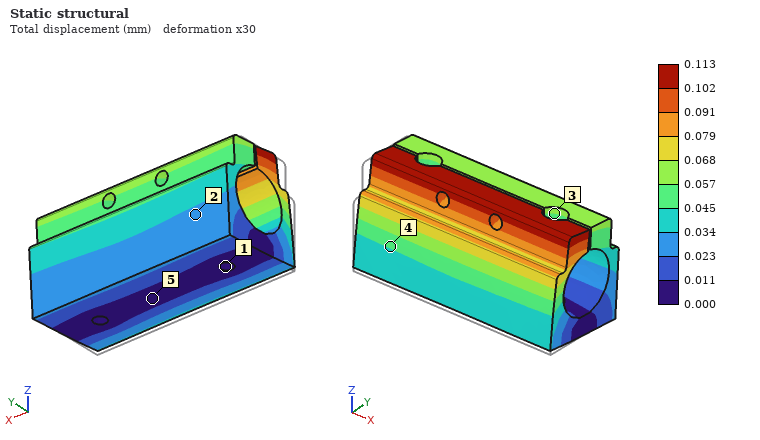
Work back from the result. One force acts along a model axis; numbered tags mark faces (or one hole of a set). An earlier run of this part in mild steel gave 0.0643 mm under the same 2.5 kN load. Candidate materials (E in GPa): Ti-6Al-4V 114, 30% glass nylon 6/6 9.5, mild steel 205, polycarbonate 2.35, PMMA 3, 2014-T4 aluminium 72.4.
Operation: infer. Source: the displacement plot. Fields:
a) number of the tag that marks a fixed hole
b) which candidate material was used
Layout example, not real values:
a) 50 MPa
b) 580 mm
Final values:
a) 1
b) Ti-6Al-4V
